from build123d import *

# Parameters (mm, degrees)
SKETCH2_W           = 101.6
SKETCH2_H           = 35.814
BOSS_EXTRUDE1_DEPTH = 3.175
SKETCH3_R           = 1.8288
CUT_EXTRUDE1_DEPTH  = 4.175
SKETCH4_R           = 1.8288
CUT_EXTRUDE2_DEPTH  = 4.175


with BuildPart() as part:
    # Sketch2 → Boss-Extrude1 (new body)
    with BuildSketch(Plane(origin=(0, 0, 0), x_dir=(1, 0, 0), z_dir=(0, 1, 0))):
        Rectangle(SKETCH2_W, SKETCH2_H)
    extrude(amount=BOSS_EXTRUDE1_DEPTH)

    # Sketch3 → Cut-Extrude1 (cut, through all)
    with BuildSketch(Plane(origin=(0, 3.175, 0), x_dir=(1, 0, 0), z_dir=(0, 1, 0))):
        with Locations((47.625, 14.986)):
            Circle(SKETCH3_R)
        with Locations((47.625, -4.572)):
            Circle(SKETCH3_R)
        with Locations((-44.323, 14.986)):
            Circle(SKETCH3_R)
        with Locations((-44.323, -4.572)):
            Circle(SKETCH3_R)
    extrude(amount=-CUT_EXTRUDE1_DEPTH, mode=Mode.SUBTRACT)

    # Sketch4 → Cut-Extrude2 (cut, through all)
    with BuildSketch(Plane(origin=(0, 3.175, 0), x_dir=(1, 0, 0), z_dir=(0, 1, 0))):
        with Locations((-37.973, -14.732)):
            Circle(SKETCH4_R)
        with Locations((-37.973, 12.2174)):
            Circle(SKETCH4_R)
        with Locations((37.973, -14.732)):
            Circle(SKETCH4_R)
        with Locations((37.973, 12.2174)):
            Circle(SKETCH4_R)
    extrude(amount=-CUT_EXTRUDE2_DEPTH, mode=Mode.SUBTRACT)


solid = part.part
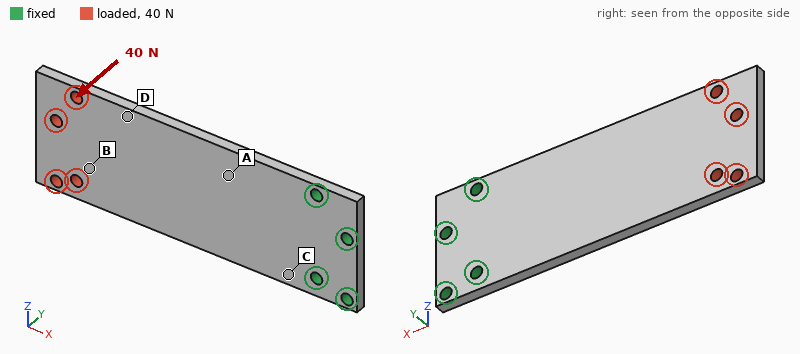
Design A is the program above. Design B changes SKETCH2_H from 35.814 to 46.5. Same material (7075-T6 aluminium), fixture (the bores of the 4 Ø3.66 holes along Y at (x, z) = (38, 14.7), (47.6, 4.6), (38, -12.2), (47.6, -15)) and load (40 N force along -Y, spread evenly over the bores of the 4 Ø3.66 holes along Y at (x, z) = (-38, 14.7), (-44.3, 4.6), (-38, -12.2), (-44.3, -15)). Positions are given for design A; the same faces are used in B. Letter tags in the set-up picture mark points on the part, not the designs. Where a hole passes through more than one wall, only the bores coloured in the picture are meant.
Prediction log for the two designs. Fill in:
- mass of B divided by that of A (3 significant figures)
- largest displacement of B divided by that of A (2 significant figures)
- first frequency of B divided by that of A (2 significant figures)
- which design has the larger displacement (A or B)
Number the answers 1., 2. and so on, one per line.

1. 1.31
2. 0.76
3. 1.0
4. A
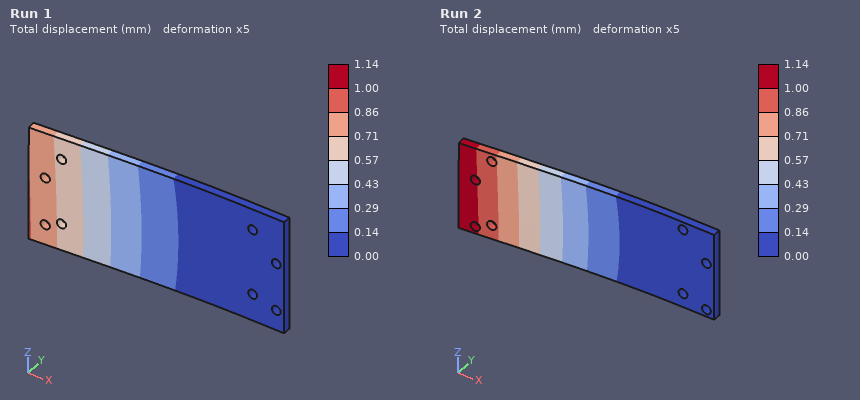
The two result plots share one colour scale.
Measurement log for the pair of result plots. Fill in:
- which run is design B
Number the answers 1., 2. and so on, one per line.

1. Run 1
